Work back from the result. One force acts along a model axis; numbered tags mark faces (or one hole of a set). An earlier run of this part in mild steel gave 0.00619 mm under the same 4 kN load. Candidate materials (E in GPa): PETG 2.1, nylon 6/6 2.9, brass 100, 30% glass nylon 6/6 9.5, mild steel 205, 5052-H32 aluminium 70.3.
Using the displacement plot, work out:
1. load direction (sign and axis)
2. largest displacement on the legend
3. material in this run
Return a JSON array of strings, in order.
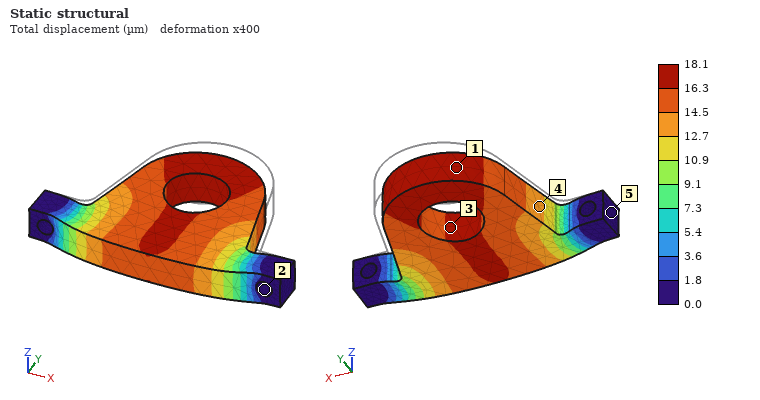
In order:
["-Y", "18.1 µm", "5052-H32 aluminium"]
